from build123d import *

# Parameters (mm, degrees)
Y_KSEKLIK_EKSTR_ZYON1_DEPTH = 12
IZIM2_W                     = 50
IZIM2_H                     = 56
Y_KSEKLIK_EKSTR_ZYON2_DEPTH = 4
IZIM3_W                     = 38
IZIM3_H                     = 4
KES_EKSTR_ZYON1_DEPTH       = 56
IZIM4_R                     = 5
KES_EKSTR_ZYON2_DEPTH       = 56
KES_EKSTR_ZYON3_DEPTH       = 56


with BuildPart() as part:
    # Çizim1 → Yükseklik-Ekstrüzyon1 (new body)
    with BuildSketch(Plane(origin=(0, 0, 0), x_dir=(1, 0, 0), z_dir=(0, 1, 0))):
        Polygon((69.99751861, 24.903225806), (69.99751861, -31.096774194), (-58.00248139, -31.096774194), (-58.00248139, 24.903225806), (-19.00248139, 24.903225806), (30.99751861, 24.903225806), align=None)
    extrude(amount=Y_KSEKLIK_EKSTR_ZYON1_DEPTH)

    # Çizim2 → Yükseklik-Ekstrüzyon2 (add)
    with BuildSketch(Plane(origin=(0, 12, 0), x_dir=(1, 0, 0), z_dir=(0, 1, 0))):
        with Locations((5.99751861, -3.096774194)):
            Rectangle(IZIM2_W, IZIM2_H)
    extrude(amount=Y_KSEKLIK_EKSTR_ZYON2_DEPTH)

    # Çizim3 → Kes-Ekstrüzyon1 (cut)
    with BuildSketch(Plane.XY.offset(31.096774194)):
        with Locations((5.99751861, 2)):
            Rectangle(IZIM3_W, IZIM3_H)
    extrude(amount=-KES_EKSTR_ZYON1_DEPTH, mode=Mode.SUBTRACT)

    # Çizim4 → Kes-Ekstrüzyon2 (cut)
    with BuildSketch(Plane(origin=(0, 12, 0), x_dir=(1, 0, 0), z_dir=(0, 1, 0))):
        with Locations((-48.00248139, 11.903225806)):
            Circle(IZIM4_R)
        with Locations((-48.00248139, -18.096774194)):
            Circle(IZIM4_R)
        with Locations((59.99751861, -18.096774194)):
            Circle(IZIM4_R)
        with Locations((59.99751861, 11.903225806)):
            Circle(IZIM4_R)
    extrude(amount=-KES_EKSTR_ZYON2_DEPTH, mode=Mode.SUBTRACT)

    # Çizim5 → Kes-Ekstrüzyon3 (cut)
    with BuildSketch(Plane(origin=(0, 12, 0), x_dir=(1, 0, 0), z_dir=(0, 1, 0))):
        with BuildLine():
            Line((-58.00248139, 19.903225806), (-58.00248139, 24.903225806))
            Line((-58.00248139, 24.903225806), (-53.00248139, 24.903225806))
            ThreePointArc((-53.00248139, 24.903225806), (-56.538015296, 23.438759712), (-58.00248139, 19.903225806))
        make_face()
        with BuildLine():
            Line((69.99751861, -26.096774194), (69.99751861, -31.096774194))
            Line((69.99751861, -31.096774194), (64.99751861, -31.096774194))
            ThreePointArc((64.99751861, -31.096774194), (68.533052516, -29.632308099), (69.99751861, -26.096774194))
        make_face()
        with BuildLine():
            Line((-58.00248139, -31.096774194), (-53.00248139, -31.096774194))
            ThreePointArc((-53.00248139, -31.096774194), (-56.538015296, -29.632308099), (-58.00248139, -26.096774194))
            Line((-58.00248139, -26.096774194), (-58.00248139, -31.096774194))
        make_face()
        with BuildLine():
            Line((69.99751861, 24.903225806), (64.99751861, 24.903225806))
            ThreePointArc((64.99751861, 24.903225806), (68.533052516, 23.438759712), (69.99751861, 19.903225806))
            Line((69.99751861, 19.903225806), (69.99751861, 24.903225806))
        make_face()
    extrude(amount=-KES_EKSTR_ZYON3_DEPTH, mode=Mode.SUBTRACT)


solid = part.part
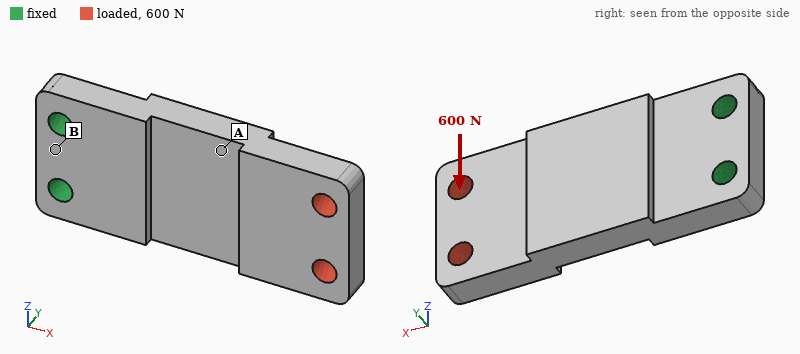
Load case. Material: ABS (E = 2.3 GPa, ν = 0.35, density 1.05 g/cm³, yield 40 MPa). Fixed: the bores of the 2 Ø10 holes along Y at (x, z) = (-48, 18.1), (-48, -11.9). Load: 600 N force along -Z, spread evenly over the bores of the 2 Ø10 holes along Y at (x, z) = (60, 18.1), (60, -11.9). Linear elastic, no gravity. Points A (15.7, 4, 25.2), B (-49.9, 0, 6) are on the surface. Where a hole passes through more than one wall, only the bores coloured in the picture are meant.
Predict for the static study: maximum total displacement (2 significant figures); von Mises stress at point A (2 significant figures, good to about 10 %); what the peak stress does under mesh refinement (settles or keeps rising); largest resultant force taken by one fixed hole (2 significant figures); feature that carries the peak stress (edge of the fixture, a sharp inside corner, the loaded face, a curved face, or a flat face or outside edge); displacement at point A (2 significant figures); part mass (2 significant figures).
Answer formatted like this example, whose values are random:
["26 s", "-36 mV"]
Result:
["1.1 mm", "5.4 MPa", "keeps rising", "1.8 kN", "edge of the fixture", "0.49 mm", "89 g"]
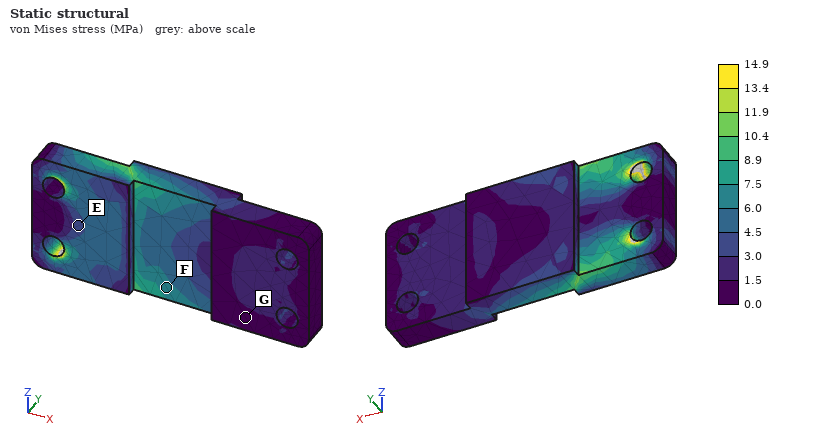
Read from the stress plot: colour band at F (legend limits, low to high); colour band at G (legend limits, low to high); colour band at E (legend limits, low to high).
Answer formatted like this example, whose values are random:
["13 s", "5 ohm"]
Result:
["6.0 to 7.5 MPa", "0.0 to 1.5 MPa", "3.0 to 4.5 MPa"]
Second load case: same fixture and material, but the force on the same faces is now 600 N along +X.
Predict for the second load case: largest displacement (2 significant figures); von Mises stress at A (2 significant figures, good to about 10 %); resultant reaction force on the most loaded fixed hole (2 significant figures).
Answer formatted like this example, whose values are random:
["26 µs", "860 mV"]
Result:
["0.39 mm", "2.6 MPa", "300 N"]
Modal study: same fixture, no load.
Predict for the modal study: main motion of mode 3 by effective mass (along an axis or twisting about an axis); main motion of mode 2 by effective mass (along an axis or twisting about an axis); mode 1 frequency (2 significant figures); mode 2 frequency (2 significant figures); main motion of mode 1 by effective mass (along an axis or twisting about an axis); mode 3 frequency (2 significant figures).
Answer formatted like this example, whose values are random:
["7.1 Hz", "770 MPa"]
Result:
["along Z", "along Z", "220 Hz", "750 Hz", "along Y", "930 Hz"]
